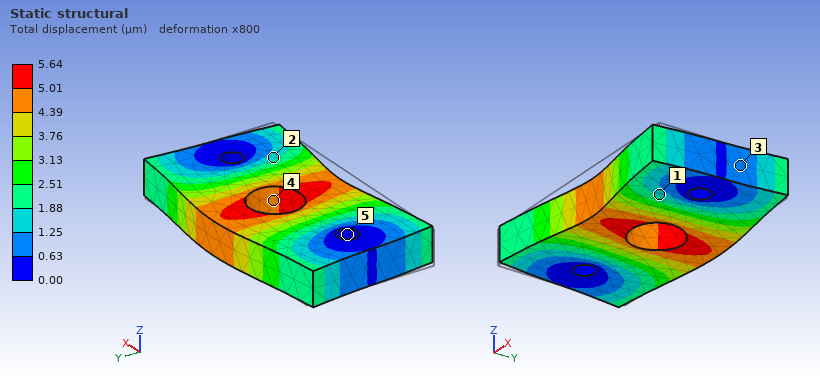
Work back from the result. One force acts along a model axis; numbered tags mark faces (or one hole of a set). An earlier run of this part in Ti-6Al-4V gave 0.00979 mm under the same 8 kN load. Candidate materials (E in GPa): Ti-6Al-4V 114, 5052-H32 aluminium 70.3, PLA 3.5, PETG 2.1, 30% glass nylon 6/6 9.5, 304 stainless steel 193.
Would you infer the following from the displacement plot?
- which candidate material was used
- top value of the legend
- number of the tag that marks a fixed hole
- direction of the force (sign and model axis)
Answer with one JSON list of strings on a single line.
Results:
["304 stainless steel", "5.64 µm", "5", "+Y"]
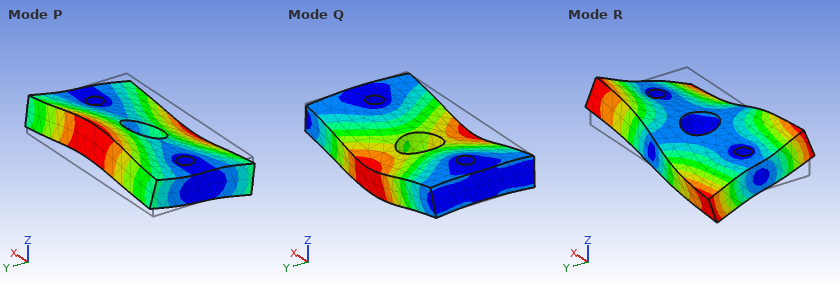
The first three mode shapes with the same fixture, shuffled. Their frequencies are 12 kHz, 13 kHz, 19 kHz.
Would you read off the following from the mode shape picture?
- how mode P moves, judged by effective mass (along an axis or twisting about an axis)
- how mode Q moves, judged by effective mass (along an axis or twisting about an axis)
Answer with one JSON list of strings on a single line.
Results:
["twisting about X", "along Z"]
